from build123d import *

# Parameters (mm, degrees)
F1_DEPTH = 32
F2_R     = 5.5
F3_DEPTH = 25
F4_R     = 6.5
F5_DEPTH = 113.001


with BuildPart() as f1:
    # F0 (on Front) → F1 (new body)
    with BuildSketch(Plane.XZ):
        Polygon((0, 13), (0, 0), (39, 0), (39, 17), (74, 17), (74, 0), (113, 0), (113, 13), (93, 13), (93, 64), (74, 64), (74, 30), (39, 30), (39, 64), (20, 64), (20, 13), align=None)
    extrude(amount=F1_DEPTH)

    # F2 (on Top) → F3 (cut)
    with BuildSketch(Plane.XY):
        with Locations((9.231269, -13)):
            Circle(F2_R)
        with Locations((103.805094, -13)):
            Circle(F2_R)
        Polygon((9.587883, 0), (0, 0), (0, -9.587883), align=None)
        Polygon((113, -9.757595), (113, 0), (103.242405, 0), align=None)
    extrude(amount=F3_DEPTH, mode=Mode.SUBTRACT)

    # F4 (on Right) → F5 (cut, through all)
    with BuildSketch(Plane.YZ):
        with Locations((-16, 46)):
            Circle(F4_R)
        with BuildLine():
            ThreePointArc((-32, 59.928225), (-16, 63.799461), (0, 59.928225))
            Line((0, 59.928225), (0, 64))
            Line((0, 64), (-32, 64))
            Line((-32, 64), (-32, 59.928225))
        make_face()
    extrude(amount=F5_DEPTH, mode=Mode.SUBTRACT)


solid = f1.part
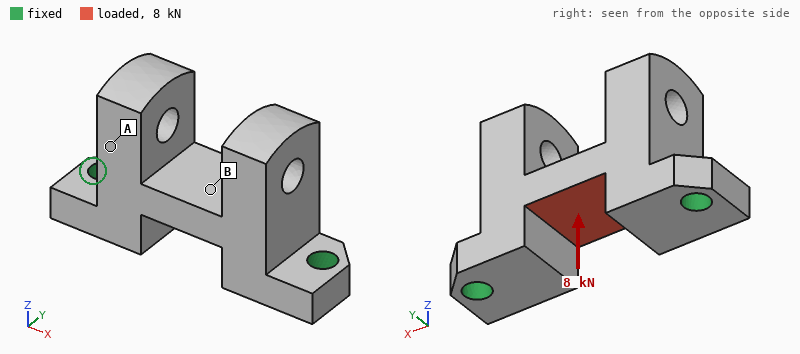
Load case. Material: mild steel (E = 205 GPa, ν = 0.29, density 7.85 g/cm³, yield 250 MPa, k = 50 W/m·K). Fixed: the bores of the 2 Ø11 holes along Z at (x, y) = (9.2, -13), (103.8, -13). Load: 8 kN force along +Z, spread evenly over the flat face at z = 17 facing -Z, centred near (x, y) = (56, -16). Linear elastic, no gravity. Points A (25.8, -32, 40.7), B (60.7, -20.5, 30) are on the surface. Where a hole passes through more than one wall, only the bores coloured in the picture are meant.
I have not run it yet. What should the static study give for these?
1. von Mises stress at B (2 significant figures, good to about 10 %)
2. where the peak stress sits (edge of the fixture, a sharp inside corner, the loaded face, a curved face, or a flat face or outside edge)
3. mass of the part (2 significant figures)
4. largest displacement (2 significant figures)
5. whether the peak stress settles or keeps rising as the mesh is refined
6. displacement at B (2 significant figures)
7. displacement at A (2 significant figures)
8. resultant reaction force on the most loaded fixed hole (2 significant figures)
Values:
38 MPa
edge of the fixture
770 g
13 µm
keeps rising
11 µm
7.5 µm
6.3 kN
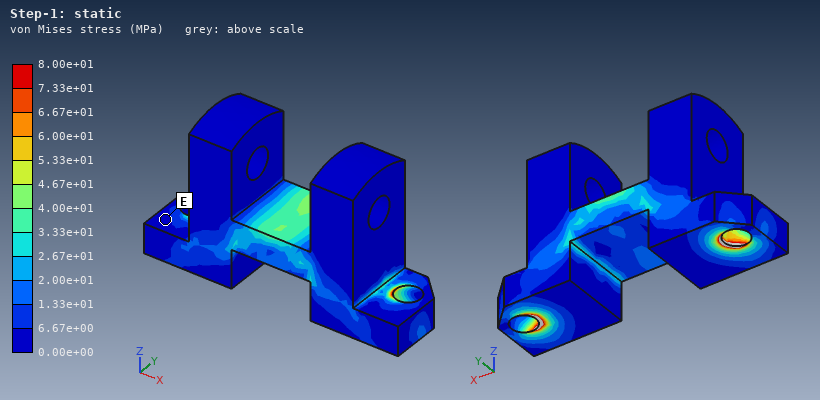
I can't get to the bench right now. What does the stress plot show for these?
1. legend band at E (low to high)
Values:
0.00e+00 to 6.67e+00 MPa
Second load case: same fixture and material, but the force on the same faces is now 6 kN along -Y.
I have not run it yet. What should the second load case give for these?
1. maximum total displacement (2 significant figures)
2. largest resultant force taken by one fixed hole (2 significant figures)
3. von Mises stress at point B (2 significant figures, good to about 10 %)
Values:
20 µm
3.0 kN
7.5 MPa
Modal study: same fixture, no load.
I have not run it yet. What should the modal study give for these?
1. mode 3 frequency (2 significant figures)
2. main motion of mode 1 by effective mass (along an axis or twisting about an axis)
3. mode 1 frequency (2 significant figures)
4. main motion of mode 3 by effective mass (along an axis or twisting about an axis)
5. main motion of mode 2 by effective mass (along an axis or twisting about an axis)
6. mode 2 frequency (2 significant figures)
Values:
5500 Hz
along Y
2900 Hz
along X
twisting about Z
4500 Hz
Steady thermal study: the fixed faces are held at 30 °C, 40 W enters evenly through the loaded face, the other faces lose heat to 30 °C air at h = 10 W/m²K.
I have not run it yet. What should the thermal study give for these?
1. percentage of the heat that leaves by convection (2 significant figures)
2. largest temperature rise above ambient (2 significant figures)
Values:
8.4 %
35 K
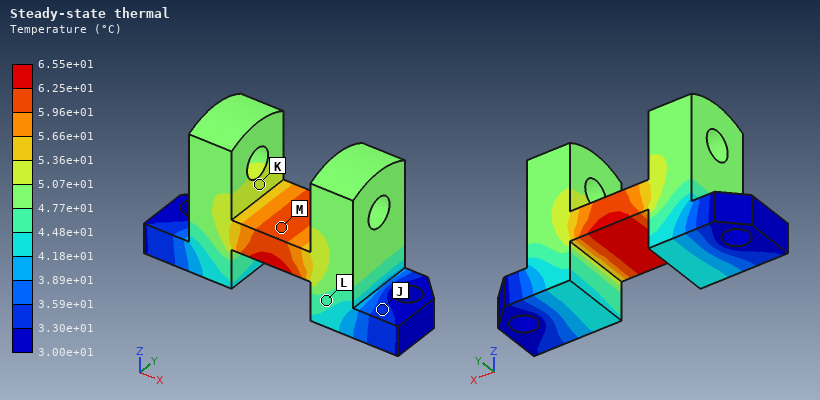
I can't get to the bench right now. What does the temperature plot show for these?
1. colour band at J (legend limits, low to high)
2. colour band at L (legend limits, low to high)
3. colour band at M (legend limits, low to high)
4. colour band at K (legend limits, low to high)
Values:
3.30e+01 to 3.59e+01 °C
4.48e+01 to 4.77e+01 °C
5.96e+01 to 6.25e+01 °C
5.07e+01 to 5.36e+01 °C
